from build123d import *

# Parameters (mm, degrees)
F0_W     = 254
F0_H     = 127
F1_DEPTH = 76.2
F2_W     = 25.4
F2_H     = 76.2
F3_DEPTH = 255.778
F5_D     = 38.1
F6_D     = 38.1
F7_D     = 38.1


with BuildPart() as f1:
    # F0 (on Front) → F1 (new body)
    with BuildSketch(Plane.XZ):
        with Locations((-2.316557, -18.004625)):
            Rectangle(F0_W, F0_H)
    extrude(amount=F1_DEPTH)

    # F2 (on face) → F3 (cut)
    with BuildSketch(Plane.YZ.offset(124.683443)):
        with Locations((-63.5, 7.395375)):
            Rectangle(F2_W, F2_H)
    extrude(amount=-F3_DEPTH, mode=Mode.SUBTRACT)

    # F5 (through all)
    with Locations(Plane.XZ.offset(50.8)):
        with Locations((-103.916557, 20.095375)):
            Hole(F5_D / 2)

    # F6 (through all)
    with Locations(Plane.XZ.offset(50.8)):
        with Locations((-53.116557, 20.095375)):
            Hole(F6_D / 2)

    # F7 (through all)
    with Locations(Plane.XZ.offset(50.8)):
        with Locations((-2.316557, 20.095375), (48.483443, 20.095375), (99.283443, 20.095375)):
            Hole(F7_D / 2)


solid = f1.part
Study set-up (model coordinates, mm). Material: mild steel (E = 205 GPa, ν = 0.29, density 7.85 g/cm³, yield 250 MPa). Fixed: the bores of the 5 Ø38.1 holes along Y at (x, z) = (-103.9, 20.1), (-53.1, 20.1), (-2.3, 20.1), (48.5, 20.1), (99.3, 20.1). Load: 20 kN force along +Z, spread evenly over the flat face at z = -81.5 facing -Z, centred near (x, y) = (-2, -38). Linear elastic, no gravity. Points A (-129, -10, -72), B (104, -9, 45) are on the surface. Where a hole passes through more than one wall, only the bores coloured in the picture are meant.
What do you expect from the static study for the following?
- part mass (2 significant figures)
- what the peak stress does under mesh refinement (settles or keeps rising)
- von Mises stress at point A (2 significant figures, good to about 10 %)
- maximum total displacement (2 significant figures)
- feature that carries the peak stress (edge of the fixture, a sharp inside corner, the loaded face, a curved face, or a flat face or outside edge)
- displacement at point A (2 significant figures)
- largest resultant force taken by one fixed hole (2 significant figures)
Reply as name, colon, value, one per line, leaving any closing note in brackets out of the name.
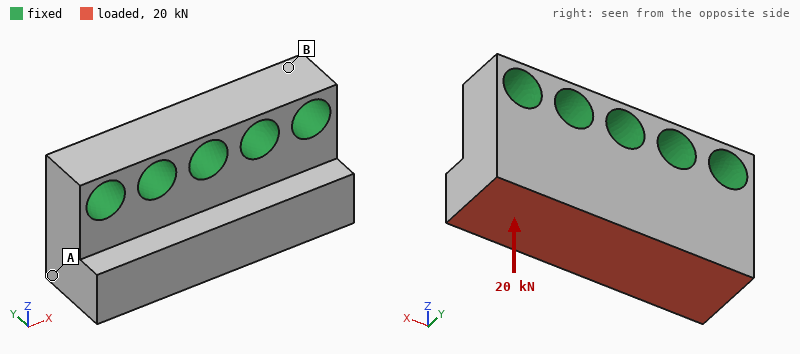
part mass: 13 kg
what the peak stress does under mesh refinement: keeps rising
von Mises stress at point A: 1.0 MPa
maximum total displacement: 2.3 µm
feature that carries the peak stress: edge of the fixture
displacement at point A: 1.1 µm
largest resultant force taken by one fixed hole: 4.4 kN
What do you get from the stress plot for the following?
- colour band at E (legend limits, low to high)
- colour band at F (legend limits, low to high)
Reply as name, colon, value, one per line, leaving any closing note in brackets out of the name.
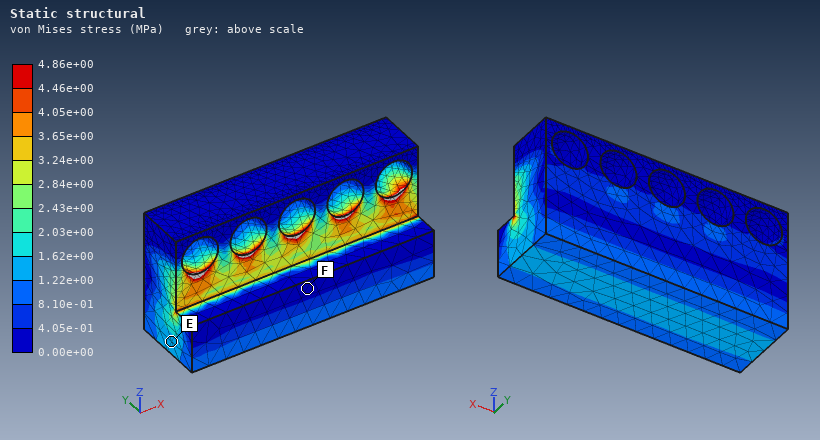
colour band at E: 1.22e+00 to 1.62e+00 MPa
colour band at F: 0.00e+00 to 4.05e-01 MPa
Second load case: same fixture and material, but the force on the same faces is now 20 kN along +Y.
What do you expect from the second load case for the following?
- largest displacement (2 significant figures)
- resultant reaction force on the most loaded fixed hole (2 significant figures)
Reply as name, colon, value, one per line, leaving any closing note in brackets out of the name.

largest displacement: 11 µm
resultant reaction force on the most loaded fixed hole: 4.3 kN
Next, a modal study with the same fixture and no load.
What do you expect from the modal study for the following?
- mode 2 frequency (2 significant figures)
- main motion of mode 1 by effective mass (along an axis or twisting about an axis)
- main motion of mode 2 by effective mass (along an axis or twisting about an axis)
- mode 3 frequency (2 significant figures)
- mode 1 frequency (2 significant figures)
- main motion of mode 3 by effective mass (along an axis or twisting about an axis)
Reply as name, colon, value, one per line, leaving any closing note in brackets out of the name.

mode 2 frequency: 4600 Hz
main motion of mode 1 by effective mass: along Y
main motion of mode 2 by effective mass: twisting about Z
mode 3 frequency: 6700 Hz
mode 1 frequency: 3600 Hz
main motion of mode 3 by effective mass: along X
